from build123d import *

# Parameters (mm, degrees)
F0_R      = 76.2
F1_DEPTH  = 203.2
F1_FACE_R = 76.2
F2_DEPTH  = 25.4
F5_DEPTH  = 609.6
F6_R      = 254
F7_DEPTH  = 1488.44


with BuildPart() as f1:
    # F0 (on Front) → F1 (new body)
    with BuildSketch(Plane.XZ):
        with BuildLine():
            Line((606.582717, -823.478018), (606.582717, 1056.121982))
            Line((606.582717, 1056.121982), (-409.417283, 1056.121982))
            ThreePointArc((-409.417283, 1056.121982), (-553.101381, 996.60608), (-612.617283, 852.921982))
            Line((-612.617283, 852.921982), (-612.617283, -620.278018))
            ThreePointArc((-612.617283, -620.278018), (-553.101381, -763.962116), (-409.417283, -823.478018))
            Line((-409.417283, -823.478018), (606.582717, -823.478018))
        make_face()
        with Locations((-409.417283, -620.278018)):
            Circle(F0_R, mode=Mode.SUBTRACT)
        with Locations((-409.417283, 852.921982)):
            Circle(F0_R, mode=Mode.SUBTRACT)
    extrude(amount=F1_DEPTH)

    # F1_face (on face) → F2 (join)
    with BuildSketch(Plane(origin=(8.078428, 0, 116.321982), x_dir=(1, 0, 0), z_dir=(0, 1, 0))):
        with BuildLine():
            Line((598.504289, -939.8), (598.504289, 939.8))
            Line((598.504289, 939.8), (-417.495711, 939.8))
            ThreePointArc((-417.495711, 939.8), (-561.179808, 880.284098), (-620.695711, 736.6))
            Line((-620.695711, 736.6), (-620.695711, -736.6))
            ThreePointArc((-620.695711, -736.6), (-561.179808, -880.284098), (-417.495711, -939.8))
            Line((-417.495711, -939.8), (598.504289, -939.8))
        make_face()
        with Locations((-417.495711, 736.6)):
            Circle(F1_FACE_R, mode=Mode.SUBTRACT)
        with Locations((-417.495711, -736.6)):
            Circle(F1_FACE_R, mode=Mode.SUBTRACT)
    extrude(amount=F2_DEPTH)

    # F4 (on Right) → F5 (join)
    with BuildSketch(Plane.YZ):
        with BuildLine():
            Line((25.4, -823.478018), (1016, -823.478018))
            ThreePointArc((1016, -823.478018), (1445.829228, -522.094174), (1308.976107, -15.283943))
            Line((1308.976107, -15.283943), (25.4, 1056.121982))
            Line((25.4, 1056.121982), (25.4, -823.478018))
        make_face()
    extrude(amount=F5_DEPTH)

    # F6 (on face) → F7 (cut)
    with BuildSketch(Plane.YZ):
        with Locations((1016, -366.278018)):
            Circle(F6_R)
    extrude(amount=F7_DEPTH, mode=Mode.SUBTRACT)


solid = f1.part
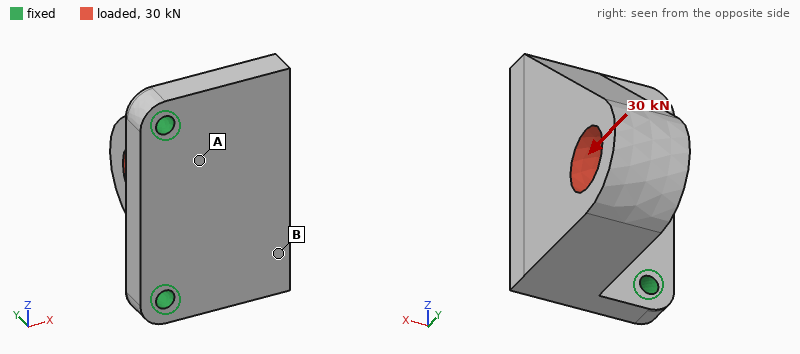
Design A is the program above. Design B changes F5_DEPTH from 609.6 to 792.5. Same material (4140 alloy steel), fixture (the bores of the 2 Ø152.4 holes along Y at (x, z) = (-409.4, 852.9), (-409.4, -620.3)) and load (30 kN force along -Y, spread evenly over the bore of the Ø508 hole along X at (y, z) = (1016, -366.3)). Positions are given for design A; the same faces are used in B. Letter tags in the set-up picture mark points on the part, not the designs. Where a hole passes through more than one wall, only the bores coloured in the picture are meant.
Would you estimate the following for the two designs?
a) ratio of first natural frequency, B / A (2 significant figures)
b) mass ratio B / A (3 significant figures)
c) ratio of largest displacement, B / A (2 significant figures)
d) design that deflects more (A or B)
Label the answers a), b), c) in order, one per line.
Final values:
a) 0.83
b) 1.20
c) 1.2
d) B
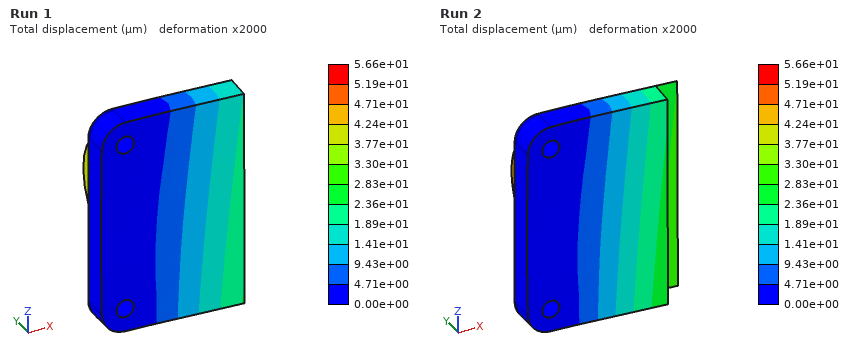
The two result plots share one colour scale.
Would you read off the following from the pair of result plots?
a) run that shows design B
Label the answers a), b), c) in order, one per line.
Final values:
a) Run 2
